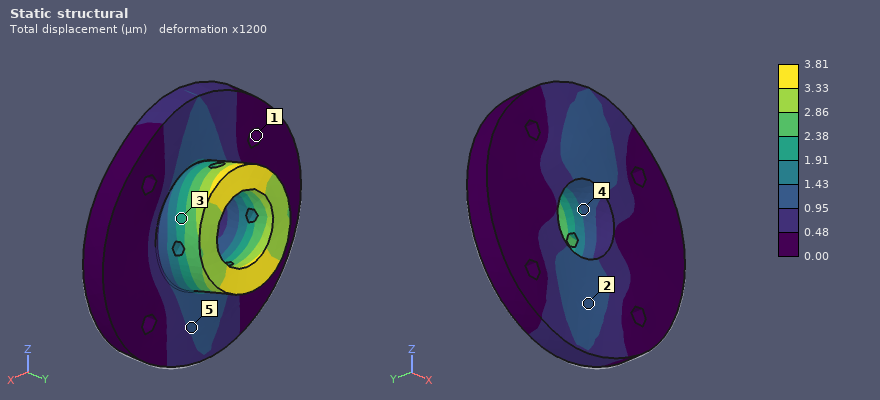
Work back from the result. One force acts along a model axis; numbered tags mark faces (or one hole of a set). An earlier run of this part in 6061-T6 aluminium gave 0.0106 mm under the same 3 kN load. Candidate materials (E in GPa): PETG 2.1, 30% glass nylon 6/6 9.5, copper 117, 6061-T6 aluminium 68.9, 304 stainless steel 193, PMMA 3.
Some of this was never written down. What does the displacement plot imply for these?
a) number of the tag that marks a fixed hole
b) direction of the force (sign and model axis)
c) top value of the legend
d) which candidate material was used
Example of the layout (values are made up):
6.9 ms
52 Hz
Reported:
1
+Z
3.81 µm
304 stainless steel
